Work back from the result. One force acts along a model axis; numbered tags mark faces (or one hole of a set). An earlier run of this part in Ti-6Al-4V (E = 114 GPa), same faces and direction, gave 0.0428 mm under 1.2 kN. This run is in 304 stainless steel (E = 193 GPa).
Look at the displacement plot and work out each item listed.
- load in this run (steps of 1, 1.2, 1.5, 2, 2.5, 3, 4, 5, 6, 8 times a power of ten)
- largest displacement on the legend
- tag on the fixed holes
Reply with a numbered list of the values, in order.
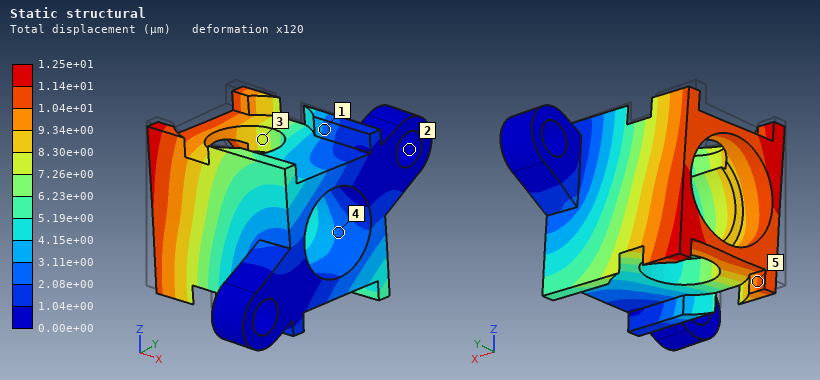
1. 600 N
2. 1.25e+01 µm
3. 2
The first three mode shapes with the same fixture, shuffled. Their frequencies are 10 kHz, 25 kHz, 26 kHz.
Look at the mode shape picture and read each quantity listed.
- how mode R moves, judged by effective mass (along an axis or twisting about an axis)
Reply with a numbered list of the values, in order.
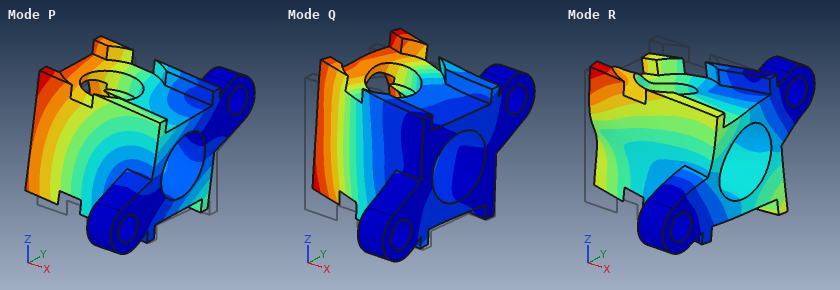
1. along X
